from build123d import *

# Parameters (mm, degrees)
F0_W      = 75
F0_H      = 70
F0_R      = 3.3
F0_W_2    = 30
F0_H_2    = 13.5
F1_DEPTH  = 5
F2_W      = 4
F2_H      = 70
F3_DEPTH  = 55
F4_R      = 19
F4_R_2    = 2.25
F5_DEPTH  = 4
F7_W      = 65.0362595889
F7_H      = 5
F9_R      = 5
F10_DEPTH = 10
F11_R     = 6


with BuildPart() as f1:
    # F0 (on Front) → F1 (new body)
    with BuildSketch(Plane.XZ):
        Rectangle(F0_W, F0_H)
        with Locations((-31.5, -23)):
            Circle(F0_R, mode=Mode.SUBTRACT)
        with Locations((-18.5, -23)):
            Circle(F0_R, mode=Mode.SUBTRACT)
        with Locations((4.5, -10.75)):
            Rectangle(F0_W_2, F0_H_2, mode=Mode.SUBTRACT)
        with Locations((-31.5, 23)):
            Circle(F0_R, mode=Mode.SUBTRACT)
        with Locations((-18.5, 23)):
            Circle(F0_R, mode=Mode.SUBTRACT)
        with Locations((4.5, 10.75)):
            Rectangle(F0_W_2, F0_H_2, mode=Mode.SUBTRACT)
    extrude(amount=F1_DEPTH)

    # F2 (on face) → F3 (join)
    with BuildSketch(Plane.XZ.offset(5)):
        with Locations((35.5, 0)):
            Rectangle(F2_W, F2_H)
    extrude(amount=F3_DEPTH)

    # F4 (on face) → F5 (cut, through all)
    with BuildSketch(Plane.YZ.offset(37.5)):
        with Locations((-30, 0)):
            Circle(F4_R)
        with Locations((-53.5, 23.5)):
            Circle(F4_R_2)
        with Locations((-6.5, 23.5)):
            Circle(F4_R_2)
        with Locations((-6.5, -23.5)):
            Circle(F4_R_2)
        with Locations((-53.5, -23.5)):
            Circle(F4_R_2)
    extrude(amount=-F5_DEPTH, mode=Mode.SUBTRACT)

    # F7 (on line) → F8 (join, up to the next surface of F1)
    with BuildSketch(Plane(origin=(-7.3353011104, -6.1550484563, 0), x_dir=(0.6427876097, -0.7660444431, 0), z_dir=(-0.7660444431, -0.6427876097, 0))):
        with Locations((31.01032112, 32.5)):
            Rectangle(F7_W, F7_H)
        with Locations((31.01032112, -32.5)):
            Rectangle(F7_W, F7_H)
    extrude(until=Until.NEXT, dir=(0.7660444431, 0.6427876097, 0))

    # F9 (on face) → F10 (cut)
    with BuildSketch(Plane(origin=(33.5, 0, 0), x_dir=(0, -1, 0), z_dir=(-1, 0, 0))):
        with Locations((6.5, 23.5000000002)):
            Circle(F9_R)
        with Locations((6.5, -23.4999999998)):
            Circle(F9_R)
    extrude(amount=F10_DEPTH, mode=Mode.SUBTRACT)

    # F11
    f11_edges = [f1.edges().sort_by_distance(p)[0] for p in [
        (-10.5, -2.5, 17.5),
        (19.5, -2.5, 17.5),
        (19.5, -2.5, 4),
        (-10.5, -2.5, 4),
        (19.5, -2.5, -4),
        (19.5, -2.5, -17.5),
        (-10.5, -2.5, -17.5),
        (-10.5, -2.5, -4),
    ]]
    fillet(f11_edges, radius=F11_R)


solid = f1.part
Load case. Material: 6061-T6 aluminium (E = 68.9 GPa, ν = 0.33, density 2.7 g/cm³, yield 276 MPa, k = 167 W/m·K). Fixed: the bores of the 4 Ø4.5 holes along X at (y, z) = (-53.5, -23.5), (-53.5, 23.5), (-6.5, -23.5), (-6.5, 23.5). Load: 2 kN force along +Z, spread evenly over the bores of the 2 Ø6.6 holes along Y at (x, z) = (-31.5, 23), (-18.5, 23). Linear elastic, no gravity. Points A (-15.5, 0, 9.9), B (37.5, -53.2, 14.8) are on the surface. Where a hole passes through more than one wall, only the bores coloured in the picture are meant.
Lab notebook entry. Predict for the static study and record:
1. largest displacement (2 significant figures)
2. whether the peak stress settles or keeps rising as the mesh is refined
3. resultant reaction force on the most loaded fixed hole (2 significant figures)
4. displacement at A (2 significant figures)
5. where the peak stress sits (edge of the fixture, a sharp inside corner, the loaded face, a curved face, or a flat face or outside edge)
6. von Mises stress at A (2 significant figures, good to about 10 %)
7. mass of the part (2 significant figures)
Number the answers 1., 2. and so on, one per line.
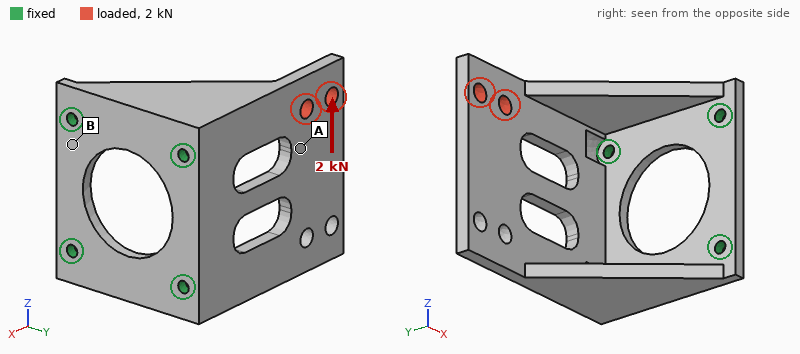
1. 0.14 mm
2. keeps rising
3. 2.6 kN
4. 0.092 mm
5. edge of the fixture
6. 23 MPa
7. 110 g
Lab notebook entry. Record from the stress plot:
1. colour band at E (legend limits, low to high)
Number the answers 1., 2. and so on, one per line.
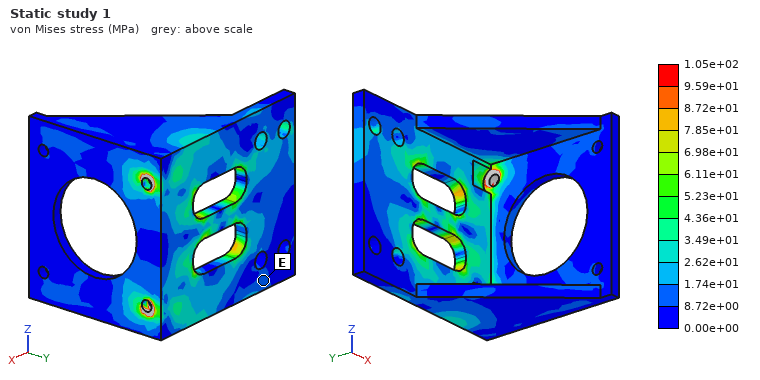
1. 8.72e+00 to 1.74e+01 MPa
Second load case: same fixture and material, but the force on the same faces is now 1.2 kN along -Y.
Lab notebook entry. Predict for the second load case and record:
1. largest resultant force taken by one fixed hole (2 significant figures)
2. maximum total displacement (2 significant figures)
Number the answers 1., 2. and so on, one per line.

1. 1.4 kN
2. 0.70 mm
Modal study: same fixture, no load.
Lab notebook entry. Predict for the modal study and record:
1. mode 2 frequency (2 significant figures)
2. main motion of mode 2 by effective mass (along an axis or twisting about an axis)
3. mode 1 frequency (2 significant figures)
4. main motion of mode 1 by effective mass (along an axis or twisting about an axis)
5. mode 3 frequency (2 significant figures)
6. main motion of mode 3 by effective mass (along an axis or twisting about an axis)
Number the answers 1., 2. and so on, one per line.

1. 3400 Hz
2. along Z
3. 1800 Hz
4. along Y
5. 4100 Hz
6. along Z
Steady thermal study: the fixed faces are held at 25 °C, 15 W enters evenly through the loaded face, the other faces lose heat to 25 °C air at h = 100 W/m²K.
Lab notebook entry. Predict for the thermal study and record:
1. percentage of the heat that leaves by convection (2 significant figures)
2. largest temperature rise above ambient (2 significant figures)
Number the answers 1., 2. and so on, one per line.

1. 53 %
2. 19 K
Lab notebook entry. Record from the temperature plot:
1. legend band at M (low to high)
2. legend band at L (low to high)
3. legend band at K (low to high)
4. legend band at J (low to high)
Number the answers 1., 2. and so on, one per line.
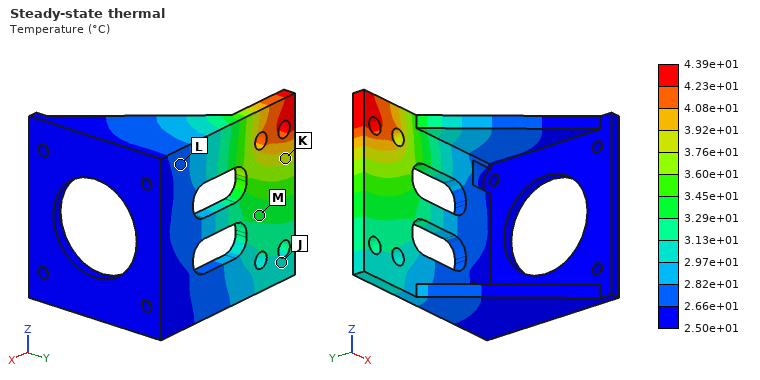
1. 3.29e+01 to 3.45e+01 °C
2. 2.66e+01 to 2.82e+01 °C
3. 3.76e+01 to 3.92e+01 °C
4. 2.97e+01 to 3.13e+01 °C
